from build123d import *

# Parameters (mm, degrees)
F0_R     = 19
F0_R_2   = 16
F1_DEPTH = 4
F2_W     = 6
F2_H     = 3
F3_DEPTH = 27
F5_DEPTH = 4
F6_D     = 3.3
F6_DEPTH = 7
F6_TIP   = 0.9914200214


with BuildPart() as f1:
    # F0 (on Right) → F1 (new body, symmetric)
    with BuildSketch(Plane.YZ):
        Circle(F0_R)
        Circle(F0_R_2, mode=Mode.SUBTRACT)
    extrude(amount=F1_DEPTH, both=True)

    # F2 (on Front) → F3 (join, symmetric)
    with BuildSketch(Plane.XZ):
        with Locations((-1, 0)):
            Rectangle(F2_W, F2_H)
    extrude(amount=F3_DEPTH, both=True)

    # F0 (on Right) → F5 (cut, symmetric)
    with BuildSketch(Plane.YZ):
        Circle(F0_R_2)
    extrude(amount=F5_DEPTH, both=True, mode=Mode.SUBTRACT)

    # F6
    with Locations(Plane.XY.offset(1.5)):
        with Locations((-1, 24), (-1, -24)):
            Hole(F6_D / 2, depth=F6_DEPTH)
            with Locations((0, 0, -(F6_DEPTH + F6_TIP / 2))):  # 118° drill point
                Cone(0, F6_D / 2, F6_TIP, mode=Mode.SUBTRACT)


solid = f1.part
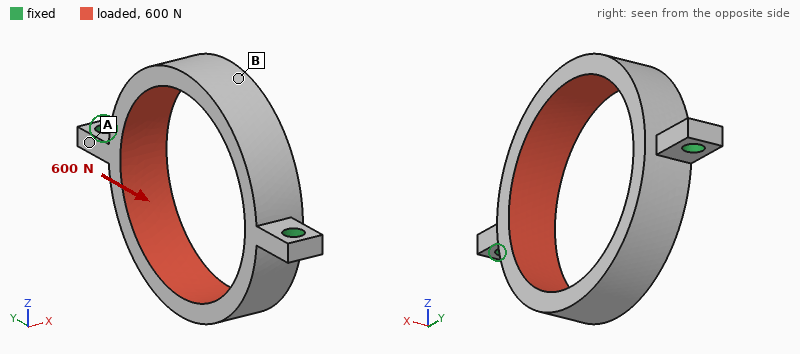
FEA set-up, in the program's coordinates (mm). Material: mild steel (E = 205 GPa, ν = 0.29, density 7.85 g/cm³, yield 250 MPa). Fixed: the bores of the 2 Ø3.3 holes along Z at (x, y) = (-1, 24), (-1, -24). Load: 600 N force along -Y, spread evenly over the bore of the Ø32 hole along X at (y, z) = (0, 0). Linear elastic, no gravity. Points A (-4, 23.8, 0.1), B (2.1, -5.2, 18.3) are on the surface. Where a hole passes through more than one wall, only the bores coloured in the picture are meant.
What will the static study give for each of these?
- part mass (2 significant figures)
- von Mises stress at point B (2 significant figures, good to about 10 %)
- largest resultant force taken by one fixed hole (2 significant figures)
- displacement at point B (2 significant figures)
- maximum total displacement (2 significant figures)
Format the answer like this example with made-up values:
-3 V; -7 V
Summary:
23 g; 15 MPa; 300 N; 7.0 µm; 8.4 µm
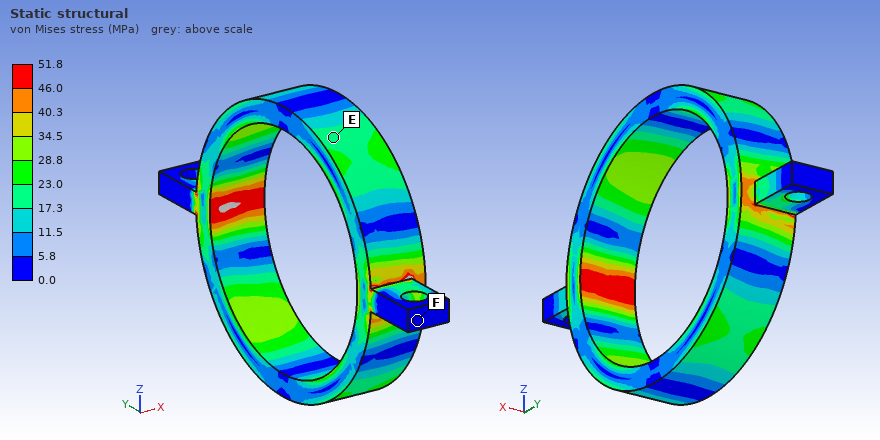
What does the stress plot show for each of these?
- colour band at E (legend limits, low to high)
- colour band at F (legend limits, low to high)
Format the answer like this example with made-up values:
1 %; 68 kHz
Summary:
17.3 to 23.0 MPa; 0.0 to 5.8 MPa
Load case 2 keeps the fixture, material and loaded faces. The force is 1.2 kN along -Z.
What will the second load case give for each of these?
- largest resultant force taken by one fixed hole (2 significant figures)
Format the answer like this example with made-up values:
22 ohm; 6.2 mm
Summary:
600 N
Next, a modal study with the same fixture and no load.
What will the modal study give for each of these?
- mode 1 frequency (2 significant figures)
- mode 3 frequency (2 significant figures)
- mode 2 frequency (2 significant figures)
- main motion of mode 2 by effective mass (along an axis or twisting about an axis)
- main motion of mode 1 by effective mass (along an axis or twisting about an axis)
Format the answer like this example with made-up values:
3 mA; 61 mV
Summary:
3300 Hz; 7100 Hz; 6800 Hz; along X; twisting about Y
